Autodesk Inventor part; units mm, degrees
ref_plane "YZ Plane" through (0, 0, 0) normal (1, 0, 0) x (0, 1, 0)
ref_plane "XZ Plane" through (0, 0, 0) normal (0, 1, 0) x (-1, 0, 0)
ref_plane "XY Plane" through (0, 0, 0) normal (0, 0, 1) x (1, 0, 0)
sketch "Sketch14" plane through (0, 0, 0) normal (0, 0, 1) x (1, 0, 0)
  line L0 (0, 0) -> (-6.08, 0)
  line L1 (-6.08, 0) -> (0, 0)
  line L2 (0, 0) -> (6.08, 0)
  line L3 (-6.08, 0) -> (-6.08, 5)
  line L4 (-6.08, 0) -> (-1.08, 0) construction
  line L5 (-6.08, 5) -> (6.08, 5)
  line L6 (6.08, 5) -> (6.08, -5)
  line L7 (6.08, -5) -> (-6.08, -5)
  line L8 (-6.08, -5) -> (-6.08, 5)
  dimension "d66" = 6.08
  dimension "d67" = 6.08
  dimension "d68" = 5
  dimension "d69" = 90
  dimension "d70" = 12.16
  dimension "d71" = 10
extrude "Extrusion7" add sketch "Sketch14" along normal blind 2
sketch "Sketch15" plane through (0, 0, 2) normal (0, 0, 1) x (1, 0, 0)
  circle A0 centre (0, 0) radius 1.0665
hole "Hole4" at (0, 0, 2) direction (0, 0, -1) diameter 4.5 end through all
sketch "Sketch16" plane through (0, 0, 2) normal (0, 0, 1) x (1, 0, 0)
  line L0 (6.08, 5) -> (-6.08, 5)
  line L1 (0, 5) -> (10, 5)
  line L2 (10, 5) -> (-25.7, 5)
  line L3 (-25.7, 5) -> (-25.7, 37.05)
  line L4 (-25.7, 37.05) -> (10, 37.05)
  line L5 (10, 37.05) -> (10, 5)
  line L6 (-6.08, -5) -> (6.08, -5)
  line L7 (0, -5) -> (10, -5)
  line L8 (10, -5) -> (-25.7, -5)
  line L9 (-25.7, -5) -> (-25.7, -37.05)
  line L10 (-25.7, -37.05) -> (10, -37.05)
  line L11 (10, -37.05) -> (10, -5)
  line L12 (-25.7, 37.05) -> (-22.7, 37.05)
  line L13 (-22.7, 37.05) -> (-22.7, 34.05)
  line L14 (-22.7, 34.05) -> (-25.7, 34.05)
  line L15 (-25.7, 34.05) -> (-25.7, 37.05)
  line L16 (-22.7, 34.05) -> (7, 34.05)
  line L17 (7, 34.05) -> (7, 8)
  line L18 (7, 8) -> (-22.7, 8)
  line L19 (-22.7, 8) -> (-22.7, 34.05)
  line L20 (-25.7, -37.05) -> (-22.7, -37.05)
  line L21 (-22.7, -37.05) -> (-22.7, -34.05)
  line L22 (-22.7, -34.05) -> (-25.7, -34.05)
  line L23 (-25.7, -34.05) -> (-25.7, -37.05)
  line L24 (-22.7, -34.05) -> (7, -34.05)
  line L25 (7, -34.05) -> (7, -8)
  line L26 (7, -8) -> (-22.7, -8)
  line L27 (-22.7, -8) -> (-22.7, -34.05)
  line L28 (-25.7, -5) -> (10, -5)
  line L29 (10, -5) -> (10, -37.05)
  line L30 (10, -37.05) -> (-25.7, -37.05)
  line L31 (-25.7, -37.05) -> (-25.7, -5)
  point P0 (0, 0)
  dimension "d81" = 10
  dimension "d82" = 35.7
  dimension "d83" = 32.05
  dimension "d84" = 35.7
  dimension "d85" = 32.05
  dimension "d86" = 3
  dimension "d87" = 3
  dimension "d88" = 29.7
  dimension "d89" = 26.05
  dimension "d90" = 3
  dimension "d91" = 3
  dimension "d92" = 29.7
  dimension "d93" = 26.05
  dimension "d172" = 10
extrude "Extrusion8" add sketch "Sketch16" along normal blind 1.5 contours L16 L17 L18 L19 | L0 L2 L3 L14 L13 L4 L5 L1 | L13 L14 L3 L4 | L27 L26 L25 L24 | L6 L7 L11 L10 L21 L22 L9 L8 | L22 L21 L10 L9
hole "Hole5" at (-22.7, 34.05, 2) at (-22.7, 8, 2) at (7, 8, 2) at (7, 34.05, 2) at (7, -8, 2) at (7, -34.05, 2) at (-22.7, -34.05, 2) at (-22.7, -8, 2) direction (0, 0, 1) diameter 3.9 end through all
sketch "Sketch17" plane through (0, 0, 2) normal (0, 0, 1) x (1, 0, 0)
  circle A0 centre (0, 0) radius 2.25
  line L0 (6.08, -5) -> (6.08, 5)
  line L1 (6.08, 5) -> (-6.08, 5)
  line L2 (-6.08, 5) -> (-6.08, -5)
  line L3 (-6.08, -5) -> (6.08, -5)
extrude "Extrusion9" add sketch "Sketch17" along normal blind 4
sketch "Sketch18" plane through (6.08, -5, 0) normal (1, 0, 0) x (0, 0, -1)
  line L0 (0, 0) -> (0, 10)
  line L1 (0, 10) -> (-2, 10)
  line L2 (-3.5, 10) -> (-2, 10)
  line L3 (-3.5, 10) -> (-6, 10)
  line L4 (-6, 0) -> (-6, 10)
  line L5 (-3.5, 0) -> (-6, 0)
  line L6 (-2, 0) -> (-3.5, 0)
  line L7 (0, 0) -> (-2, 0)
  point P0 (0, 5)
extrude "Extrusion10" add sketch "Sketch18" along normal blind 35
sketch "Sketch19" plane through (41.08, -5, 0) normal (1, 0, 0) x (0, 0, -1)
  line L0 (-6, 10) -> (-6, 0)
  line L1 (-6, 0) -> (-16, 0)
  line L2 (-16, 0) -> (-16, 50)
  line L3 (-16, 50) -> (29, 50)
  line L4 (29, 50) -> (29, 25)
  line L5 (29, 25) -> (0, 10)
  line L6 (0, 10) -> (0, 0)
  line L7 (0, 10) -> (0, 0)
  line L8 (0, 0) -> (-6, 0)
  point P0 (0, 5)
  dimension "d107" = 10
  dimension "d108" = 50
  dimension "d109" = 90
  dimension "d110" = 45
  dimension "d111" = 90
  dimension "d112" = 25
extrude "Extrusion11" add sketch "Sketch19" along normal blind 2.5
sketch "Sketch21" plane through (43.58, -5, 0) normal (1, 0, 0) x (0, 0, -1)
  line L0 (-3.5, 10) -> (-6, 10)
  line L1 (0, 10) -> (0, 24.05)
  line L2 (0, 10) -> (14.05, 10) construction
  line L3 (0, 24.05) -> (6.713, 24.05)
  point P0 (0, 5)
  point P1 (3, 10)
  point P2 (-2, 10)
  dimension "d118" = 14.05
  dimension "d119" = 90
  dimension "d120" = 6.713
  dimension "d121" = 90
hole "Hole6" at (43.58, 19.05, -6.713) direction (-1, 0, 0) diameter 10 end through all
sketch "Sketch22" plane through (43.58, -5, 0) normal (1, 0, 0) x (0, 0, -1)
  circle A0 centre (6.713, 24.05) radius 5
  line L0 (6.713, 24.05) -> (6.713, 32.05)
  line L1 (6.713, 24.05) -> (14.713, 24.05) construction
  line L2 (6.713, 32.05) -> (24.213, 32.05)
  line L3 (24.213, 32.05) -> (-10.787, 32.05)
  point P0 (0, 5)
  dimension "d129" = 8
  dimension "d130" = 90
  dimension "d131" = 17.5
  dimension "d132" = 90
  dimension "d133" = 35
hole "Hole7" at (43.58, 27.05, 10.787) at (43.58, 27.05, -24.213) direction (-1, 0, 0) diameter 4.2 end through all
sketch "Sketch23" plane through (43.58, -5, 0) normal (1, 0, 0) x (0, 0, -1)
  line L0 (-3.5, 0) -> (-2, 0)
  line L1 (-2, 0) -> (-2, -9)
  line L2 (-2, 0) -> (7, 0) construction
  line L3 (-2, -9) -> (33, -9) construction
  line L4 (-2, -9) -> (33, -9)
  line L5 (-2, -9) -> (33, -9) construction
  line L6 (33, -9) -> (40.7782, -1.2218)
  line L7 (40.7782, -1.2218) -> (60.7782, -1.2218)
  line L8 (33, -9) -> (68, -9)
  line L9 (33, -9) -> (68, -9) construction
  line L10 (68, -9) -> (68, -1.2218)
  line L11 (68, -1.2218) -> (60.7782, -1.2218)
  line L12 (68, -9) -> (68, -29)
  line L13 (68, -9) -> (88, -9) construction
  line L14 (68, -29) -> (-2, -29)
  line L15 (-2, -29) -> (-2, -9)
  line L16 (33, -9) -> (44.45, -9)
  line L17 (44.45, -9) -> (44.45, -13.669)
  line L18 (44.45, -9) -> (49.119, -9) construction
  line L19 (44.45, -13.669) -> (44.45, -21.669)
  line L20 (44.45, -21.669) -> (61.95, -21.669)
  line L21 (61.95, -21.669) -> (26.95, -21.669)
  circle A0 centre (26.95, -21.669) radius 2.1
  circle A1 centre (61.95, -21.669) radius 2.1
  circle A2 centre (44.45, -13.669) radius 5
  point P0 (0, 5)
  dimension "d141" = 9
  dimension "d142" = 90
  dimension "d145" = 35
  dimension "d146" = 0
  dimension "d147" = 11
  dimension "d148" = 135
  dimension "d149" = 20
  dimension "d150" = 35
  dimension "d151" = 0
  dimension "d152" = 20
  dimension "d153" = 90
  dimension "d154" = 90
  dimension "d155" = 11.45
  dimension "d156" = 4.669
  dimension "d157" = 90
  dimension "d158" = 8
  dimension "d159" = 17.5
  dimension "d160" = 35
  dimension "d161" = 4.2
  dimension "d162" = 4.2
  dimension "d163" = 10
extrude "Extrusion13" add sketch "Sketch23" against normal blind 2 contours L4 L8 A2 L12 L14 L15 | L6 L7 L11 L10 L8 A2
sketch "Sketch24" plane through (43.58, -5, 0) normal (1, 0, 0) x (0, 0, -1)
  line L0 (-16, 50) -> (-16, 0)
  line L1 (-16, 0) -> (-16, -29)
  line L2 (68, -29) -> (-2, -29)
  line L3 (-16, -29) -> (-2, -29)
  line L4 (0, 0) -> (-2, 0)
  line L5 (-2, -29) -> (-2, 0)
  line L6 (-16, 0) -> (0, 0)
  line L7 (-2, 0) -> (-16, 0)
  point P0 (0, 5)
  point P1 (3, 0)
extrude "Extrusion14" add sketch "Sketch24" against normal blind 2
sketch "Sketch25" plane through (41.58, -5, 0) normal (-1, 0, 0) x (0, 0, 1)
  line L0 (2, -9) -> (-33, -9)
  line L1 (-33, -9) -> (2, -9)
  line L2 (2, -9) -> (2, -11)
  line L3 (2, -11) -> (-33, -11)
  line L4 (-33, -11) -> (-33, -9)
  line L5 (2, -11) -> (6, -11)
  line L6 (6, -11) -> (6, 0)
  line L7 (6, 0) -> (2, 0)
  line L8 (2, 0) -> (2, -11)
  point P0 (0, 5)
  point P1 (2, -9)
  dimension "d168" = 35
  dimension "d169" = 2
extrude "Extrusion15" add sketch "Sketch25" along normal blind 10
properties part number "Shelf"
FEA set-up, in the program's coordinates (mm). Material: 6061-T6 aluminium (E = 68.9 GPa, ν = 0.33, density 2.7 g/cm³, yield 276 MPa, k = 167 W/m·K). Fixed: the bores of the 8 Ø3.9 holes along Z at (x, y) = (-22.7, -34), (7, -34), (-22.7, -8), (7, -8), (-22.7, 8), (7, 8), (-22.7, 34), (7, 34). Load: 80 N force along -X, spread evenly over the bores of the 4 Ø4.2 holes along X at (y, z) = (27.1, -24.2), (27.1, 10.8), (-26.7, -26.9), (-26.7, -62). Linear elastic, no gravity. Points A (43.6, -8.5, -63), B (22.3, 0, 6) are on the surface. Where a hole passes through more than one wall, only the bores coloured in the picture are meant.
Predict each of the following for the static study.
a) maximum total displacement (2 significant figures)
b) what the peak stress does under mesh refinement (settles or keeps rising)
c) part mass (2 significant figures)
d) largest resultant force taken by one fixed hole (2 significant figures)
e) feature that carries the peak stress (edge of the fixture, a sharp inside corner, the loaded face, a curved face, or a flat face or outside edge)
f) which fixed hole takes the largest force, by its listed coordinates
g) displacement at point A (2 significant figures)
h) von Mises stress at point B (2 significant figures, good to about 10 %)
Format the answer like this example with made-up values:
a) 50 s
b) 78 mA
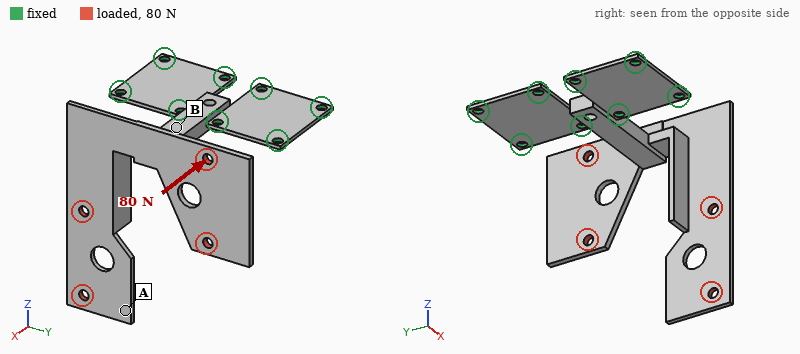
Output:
a) 1.4 mm
b) keeps rising
c) 41 g
d) 57 N
e) edge of the fixture
f) (7, 8)
g) 0.99 mm
h) 34 MPa
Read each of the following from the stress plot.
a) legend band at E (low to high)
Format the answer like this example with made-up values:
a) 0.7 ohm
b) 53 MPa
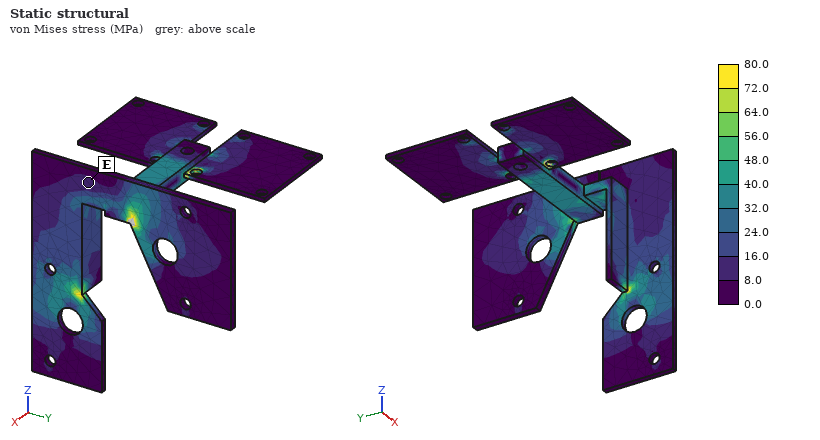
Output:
a) 8.0 to 16.0 MPa
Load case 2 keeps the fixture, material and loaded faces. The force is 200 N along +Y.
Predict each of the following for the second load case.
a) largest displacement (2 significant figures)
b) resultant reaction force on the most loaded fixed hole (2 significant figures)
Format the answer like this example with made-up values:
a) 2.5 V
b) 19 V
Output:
a) 1.5 mm
b) 620 N
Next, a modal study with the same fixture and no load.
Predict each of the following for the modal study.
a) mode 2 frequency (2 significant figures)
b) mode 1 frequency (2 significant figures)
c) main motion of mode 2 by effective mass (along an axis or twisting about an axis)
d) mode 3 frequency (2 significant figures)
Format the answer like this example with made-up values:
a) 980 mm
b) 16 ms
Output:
a) 490 Hz
b) 380 Hz
c) along Y
d) 620 Hz
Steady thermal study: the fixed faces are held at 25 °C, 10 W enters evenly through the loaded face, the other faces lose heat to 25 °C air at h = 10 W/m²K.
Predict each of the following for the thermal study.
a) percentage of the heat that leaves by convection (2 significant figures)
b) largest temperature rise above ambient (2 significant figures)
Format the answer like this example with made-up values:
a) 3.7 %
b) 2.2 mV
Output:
a) 34 %
b) 48 K
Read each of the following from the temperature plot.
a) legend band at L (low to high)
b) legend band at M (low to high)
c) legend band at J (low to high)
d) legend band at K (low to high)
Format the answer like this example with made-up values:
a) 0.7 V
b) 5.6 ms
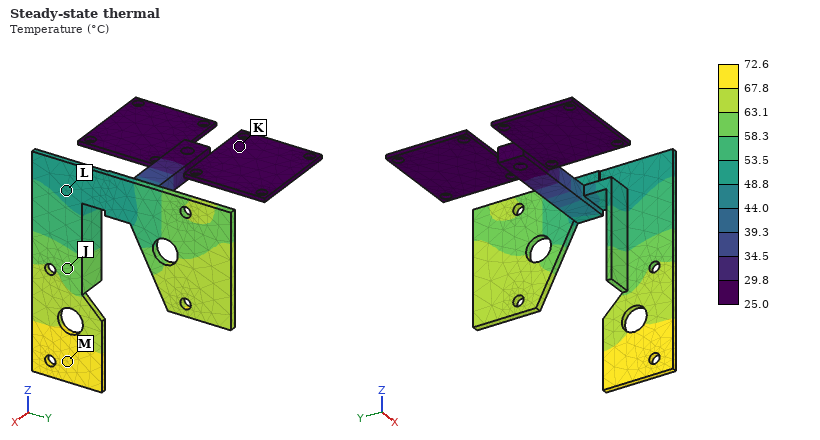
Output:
a) 48.8 to 53.5 °C
b) 67.8 to 72.6 °C
c) 58.3 to 63.1 °C
d) 25.0 to 29.8 °C
